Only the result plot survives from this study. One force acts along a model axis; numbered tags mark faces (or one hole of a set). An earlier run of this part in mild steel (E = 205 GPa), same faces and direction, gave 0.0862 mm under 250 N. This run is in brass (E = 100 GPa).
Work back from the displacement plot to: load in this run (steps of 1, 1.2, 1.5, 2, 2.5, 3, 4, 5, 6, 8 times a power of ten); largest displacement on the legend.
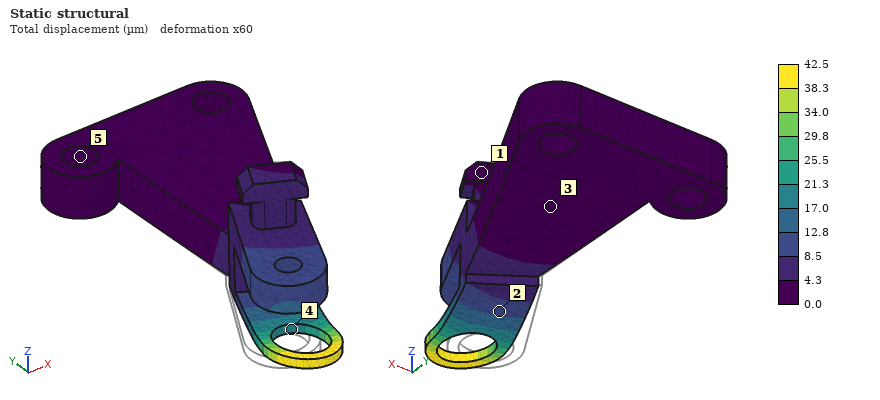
60 N
42.5 µm
